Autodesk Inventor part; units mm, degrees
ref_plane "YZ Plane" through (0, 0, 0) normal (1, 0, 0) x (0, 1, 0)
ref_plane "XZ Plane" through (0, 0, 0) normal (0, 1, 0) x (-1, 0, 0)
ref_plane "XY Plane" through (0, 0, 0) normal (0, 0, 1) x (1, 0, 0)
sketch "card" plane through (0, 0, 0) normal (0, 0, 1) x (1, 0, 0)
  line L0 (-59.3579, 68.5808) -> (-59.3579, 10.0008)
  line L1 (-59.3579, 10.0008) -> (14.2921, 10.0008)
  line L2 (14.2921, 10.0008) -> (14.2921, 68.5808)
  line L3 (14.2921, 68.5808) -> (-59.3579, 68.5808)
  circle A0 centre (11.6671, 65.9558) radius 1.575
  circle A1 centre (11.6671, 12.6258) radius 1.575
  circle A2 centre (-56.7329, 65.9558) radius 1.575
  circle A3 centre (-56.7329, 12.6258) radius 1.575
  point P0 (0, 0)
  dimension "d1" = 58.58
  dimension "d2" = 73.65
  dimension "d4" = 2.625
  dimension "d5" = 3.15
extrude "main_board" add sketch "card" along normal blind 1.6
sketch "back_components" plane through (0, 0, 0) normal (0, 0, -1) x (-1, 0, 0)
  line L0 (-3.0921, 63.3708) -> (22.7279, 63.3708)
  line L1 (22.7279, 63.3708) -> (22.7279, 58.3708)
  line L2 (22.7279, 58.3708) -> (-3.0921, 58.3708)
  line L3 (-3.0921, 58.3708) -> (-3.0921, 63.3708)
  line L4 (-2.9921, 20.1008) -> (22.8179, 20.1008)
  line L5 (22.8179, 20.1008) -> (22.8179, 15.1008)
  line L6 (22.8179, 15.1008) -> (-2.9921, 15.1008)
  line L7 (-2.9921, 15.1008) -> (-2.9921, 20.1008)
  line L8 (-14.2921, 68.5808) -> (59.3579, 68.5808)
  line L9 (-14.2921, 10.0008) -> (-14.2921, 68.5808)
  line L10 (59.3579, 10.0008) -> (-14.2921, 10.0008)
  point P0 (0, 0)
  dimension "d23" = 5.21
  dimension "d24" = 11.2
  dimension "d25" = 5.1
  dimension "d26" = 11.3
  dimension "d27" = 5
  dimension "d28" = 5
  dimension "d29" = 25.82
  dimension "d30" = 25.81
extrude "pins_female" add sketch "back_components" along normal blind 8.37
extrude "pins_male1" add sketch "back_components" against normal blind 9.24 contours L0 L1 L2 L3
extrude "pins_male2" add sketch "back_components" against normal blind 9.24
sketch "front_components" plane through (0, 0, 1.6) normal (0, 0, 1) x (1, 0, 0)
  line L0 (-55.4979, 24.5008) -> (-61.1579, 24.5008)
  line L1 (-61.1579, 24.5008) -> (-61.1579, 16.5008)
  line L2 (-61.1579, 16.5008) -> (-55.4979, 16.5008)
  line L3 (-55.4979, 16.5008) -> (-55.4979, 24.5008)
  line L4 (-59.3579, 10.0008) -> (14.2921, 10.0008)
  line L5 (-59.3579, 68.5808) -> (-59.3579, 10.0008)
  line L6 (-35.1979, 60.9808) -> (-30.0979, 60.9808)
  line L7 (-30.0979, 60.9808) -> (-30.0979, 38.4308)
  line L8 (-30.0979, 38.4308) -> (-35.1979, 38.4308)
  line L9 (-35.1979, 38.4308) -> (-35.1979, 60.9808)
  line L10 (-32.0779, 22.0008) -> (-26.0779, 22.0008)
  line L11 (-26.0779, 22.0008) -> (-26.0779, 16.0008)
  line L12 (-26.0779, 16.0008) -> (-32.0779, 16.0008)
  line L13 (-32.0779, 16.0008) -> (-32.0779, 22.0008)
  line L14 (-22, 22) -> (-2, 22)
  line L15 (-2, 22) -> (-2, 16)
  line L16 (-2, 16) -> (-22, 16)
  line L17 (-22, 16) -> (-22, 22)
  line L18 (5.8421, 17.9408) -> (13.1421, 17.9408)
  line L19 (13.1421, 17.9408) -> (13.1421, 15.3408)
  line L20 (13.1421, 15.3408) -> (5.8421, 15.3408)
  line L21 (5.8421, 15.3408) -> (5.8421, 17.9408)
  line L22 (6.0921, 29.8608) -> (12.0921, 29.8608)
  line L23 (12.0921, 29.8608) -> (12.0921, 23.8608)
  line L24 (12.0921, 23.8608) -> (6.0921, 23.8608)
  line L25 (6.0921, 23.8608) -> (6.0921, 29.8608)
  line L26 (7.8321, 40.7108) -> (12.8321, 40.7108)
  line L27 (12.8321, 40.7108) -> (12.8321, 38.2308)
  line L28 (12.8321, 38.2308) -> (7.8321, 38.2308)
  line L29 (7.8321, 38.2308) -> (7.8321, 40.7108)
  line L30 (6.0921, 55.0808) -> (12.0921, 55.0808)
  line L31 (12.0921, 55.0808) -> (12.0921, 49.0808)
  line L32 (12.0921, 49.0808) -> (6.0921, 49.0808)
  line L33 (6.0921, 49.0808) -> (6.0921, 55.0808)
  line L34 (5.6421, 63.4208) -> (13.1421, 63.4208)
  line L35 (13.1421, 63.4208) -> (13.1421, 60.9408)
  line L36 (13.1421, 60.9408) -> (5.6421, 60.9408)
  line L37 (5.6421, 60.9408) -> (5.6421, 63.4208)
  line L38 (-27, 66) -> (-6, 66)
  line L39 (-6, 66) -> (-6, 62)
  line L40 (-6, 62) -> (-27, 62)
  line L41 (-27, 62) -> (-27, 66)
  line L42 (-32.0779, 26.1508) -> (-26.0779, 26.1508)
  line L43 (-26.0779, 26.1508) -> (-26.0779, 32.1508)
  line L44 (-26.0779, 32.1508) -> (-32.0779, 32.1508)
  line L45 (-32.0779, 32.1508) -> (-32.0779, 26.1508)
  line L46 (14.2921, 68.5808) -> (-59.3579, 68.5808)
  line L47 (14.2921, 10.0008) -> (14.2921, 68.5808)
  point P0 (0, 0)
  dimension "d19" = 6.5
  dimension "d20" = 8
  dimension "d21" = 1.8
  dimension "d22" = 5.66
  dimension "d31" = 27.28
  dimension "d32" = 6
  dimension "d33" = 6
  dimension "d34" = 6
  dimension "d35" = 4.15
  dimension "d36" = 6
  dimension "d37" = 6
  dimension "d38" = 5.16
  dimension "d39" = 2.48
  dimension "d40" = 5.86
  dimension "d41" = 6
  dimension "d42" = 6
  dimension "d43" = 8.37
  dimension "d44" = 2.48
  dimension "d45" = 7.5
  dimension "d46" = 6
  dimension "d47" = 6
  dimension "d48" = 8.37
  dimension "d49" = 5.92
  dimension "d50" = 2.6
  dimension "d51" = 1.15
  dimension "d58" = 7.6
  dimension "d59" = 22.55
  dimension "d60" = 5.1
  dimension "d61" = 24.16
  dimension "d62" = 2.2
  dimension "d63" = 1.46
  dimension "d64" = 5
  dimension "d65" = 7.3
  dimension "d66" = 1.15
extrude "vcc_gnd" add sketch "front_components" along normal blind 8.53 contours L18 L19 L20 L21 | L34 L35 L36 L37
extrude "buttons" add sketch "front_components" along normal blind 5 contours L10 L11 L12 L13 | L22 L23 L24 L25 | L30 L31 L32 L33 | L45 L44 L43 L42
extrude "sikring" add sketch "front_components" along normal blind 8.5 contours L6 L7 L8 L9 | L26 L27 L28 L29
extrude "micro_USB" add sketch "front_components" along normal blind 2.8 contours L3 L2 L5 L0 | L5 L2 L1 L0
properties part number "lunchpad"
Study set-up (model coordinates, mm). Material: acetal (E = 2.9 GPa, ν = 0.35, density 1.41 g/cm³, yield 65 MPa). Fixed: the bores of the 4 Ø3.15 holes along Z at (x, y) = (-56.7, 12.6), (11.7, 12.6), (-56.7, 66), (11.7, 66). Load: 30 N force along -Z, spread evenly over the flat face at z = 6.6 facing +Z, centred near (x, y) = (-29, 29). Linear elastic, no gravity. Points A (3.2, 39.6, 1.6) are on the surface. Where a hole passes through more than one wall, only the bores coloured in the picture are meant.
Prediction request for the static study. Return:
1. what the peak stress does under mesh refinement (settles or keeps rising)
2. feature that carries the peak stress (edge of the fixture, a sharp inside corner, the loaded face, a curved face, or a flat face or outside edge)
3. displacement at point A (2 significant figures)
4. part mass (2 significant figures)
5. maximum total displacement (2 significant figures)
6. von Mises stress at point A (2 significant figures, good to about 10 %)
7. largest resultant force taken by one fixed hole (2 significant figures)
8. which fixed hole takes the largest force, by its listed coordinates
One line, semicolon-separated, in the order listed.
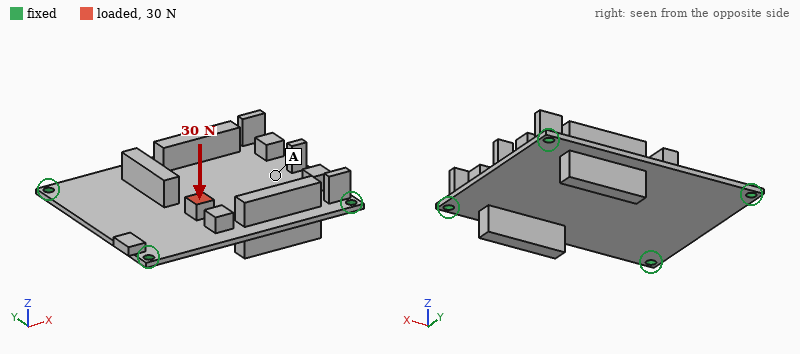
keeps rising; edge of the fixture; 0.37 mm; 19 g; 1.1 mm; 2.9 MPa; 13 N; (-56.7, 12.6)
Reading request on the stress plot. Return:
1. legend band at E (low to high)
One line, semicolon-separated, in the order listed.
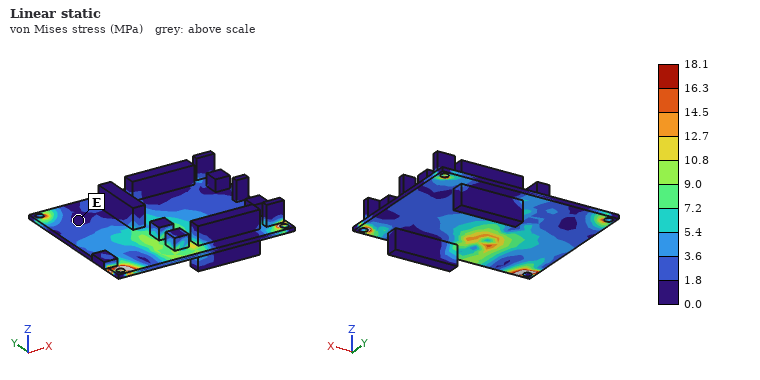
0.0 to 1.8 MPa
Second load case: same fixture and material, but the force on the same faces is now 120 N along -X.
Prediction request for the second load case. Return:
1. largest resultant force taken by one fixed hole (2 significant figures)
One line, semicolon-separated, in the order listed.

40 N
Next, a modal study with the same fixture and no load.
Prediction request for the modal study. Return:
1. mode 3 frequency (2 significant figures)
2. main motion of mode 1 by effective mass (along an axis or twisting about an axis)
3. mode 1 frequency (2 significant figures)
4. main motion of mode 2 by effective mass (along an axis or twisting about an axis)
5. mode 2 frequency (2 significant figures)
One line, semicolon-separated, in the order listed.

740 Hz; along Z; 340 Hz; twisting about X; 540 Hz
